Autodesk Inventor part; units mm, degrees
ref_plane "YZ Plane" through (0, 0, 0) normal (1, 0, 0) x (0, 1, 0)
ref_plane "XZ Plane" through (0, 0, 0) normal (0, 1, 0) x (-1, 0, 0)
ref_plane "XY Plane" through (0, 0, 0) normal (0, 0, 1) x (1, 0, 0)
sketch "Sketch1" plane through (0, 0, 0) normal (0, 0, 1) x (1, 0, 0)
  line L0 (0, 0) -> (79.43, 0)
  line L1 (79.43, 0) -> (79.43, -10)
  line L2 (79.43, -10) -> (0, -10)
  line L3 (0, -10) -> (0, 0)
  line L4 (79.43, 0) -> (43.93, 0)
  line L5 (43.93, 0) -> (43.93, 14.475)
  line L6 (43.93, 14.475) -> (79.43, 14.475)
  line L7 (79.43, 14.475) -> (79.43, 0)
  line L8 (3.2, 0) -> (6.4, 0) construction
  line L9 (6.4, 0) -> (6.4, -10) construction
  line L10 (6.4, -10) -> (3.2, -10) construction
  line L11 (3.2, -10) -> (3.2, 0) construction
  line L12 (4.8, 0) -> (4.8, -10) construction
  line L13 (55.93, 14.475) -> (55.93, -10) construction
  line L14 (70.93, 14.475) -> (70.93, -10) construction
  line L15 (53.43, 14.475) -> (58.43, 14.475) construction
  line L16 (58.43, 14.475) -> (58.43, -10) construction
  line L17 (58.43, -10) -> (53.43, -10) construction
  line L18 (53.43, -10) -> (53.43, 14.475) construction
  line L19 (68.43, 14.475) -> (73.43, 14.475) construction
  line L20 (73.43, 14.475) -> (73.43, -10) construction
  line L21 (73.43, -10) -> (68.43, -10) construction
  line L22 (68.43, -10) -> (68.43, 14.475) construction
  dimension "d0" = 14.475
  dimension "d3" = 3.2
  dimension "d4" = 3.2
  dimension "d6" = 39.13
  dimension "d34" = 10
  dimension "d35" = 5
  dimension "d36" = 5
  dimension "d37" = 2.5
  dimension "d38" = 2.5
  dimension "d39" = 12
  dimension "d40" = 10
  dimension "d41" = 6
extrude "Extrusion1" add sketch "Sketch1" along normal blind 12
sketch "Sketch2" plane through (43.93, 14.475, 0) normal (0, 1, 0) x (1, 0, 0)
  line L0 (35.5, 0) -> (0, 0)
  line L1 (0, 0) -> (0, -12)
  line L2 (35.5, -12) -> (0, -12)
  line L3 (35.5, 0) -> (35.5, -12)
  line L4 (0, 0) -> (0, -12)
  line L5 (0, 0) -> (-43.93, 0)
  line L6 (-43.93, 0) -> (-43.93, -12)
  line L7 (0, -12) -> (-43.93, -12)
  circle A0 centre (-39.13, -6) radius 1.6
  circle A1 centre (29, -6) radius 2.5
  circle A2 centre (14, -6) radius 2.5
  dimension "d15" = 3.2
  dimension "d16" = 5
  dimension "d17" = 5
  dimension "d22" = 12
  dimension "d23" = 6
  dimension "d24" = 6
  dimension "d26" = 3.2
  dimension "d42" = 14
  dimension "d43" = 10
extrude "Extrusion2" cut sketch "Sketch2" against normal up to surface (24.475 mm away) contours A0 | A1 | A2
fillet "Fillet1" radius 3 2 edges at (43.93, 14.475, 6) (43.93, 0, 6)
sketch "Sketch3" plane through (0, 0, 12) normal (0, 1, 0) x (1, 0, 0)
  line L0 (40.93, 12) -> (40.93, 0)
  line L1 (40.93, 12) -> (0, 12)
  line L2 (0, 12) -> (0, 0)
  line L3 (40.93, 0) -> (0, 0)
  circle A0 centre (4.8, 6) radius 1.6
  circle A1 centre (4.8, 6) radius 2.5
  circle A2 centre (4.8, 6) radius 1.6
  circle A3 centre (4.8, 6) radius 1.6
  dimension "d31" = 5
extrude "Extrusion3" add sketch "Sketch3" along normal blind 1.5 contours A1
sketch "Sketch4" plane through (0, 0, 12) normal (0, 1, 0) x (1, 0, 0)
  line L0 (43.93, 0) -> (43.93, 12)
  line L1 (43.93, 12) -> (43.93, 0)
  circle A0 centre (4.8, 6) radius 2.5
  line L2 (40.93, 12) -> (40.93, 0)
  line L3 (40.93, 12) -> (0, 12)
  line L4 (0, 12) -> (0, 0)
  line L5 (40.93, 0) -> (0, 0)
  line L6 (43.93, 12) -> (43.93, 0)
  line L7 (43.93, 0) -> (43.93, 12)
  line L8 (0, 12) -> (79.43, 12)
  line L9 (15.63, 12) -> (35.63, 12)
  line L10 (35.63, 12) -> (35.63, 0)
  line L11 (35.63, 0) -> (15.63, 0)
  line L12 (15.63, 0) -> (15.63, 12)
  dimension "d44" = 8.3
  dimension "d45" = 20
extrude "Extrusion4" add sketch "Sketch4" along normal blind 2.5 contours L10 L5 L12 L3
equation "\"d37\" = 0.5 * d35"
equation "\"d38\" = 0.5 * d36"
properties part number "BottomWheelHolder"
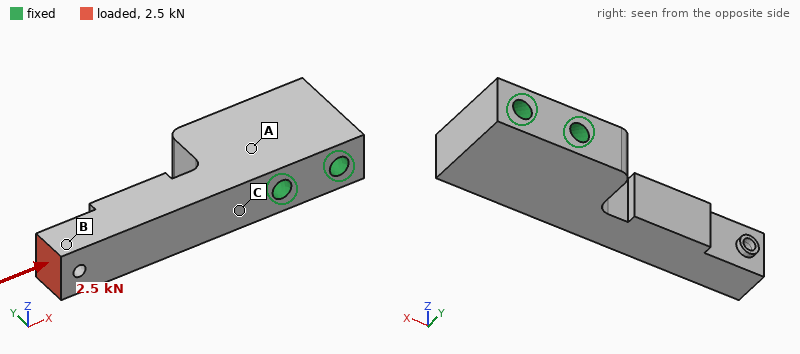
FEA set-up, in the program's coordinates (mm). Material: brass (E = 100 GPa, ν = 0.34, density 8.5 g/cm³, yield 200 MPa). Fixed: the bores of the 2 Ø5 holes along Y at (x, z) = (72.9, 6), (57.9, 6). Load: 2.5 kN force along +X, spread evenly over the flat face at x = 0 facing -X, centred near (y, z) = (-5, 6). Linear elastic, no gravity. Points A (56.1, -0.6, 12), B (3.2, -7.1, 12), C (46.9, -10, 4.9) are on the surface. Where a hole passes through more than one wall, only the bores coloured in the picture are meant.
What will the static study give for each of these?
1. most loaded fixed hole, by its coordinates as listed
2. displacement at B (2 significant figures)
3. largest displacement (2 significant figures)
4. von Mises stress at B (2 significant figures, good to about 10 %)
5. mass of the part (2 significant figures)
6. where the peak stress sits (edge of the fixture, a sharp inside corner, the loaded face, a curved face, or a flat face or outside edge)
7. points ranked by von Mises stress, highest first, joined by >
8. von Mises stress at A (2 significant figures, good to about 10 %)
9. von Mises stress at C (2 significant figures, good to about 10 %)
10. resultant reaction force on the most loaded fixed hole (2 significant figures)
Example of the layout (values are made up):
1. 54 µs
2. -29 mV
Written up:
1. (57.9, 6)
2. 20 µm
3. 23 µm
4. 17 MPa
5. 130 g
6. a curved face
7. C > B > A
8. 6.1 MPa
9. 26 MPa
10. 2.3 kN
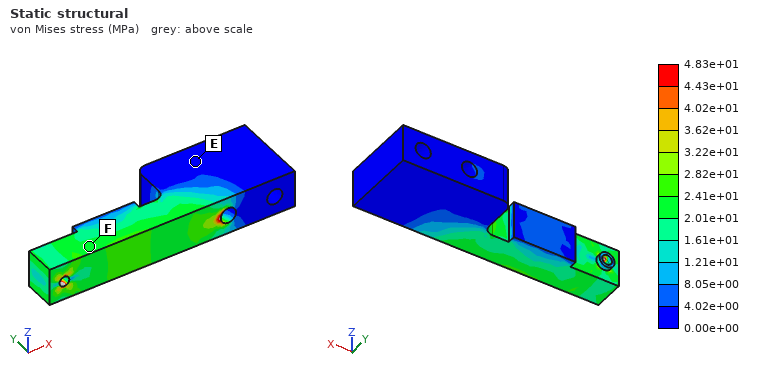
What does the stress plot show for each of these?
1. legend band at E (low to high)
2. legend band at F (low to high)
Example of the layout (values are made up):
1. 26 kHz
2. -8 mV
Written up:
1. 0.00e+00 to 4.02e+00 MPa
2. 2.01e+01 to 2.41e+01 MPa
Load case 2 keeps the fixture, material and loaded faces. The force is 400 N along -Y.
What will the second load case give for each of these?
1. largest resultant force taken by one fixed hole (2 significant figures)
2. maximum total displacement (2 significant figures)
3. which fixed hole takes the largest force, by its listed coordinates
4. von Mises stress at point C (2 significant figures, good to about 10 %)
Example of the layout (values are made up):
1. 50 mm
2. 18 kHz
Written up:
1. 450 N
2. 0.14 mm
3. (57.9, 6)
4. 59 MPa
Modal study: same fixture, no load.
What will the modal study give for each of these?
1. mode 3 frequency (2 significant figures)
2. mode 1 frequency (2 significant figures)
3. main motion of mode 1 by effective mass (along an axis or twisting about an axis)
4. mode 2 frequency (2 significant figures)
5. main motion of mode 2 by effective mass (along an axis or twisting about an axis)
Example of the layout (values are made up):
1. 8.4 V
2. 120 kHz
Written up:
1. 9500 Hz
2. 2100 Hz
3. along Z
4. 2400 Hz
5. along Y
